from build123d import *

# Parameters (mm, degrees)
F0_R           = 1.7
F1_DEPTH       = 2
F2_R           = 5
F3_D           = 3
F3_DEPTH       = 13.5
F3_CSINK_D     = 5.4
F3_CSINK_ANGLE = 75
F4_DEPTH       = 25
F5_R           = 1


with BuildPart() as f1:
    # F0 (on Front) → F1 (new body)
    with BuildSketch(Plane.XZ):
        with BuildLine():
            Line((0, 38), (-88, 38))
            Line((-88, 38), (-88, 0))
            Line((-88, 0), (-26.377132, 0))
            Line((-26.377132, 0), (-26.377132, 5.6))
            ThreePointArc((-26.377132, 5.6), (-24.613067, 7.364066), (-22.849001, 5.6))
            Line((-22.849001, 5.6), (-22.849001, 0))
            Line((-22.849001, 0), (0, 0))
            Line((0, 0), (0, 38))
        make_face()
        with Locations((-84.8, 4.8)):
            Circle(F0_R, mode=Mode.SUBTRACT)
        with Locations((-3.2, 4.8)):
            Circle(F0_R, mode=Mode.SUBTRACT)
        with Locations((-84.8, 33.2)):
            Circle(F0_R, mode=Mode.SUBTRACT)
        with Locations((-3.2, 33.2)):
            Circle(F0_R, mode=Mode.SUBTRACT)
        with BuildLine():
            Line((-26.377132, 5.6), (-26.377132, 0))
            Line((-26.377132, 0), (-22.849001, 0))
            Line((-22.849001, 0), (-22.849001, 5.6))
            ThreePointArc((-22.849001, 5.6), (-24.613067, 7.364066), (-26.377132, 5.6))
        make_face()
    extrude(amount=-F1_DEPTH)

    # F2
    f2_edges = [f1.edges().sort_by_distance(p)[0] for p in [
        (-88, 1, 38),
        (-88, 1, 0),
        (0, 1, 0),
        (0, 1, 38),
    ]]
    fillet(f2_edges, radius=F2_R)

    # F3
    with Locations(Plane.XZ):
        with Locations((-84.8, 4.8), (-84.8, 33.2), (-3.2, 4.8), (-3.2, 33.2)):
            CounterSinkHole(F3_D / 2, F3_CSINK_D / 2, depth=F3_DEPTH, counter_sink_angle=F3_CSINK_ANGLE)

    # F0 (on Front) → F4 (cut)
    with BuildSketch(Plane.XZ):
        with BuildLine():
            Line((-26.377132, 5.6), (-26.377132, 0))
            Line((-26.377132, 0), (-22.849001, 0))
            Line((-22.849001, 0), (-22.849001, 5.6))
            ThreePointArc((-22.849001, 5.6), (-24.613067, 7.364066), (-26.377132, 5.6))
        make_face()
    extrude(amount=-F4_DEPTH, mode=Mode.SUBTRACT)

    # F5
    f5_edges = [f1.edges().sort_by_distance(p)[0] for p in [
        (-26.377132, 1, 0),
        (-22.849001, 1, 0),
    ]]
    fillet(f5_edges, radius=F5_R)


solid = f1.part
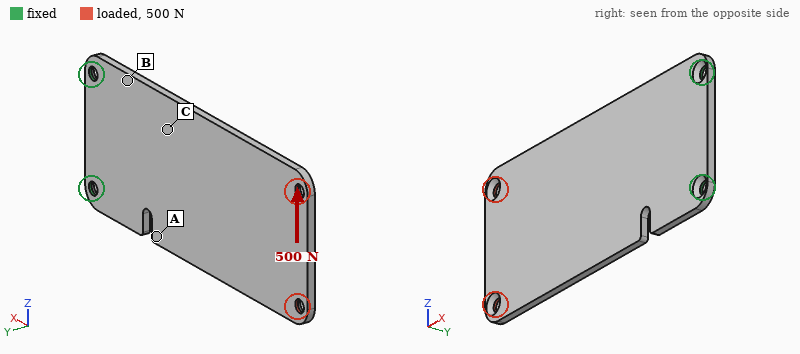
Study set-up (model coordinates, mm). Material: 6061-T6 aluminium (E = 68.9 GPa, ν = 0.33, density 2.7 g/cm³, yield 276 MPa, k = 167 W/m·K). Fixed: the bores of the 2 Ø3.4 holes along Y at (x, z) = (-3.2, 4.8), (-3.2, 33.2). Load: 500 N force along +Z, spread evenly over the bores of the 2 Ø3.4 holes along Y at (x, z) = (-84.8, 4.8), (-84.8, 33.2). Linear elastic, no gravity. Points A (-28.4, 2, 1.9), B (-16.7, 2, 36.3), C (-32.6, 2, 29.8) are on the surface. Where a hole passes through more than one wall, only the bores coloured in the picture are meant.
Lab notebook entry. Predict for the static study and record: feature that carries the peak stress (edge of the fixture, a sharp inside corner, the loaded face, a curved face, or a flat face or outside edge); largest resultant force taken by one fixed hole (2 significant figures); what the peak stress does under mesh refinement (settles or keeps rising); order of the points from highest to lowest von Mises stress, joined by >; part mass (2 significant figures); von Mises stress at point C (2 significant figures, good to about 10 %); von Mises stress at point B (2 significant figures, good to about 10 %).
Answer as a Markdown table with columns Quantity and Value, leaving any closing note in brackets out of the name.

| Quantity | Value |
|---|---|
| feature that carries the peak stress | edge of the fixture |
| largest resultant force taken by one fixed hole | 1.4 kN |
| what the peak stress does under mesh refinement | keeps rising |
| order of the points from highest to lowest von Mises stress, joined by > | B > C > A |
| part mass | 18 g |
| von Mises stress at point C | 48 MPa |
| von Mises stress at point B | 86 MPa |
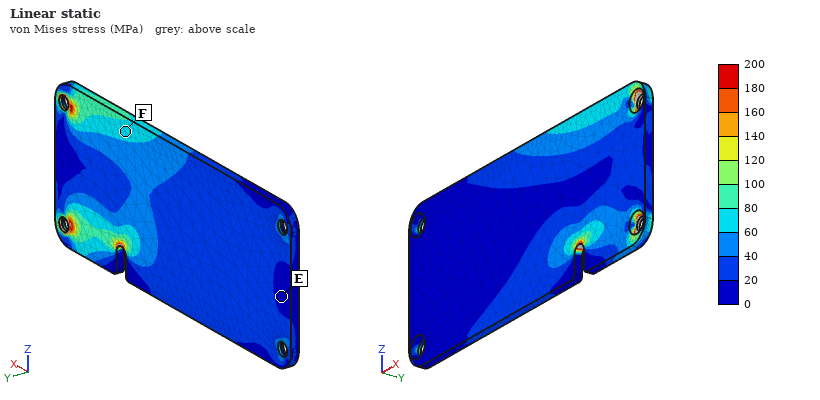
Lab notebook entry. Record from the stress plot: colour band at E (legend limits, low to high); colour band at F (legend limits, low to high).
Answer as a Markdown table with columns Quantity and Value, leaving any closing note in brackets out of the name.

| Quantity | Value |
|---|---|
| colour band at E | 0 to 20 MPa |
| colour band at F | 60 to 80 MPa |
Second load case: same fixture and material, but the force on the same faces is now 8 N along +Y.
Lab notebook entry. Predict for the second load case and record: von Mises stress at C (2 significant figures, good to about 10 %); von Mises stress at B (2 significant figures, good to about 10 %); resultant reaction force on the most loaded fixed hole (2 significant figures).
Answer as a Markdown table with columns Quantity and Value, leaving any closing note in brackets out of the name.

| Quantity | Value |
|---|---|
| von Mises stress at C | 18 MPa |
| von Mises stress at B | 24 MPa |
| resultant reaction force on the most loaded fixed hole | 4.8 N |
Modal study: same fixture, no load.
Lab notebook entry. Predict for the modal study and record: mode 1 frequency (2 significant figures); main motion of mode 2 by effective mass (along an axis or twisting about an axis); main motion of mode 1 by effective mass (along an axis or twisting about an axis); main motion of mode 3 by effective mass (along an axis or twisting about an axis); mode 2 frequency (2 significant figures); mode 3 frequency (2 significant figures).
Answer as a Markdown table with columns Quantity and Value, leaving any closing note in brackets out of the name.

| Quantity | Value |
|---|---|
| mode 1 frequency | 200 Hz |
| main motion of mode 2 by effective mass | twisting about X |
| main motion of mode 1 by effective mass | along Y |
| main motion of mode 3 by effective mass | along Y |
| mode 2 frequency | 1000 Hz |
| mode 3 frequency | 1300 Hz |
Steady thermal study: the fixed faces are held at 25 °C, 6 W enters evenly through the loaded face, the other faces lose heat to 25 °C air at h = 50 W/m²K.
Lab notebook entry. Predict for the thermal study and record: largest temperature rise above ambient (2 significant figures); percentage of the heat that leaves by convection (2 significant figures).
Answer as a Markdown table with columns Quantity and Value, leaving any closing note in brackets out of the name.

| Quantity | Value |
|---|---|
| largest temperature rise above ambient | 28 K |
| percentage of the heat that leaves by convection | 63 % |
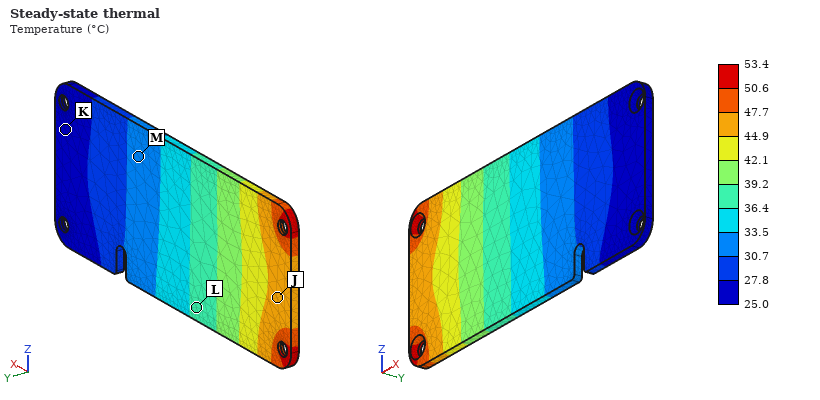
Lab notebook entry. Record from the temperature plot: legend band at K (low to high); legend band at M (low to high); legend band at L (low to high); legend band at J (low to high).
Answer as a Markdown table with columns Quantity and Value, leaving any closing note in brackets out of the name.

| Quantity | Value |
|---|---|
| legend band at K | 25.0 to 27.8 °C |
| legend band at M | 30.7 to 33.5 °C |
| legend band at L | 36.4 to 39.2 °C |
| legend band at J | 44.9 to 47.7 °C |
